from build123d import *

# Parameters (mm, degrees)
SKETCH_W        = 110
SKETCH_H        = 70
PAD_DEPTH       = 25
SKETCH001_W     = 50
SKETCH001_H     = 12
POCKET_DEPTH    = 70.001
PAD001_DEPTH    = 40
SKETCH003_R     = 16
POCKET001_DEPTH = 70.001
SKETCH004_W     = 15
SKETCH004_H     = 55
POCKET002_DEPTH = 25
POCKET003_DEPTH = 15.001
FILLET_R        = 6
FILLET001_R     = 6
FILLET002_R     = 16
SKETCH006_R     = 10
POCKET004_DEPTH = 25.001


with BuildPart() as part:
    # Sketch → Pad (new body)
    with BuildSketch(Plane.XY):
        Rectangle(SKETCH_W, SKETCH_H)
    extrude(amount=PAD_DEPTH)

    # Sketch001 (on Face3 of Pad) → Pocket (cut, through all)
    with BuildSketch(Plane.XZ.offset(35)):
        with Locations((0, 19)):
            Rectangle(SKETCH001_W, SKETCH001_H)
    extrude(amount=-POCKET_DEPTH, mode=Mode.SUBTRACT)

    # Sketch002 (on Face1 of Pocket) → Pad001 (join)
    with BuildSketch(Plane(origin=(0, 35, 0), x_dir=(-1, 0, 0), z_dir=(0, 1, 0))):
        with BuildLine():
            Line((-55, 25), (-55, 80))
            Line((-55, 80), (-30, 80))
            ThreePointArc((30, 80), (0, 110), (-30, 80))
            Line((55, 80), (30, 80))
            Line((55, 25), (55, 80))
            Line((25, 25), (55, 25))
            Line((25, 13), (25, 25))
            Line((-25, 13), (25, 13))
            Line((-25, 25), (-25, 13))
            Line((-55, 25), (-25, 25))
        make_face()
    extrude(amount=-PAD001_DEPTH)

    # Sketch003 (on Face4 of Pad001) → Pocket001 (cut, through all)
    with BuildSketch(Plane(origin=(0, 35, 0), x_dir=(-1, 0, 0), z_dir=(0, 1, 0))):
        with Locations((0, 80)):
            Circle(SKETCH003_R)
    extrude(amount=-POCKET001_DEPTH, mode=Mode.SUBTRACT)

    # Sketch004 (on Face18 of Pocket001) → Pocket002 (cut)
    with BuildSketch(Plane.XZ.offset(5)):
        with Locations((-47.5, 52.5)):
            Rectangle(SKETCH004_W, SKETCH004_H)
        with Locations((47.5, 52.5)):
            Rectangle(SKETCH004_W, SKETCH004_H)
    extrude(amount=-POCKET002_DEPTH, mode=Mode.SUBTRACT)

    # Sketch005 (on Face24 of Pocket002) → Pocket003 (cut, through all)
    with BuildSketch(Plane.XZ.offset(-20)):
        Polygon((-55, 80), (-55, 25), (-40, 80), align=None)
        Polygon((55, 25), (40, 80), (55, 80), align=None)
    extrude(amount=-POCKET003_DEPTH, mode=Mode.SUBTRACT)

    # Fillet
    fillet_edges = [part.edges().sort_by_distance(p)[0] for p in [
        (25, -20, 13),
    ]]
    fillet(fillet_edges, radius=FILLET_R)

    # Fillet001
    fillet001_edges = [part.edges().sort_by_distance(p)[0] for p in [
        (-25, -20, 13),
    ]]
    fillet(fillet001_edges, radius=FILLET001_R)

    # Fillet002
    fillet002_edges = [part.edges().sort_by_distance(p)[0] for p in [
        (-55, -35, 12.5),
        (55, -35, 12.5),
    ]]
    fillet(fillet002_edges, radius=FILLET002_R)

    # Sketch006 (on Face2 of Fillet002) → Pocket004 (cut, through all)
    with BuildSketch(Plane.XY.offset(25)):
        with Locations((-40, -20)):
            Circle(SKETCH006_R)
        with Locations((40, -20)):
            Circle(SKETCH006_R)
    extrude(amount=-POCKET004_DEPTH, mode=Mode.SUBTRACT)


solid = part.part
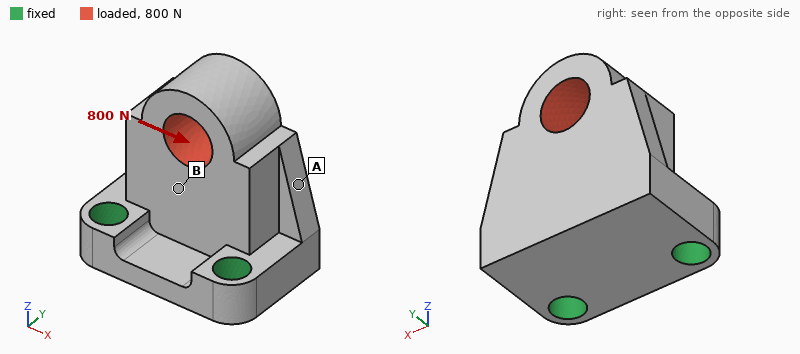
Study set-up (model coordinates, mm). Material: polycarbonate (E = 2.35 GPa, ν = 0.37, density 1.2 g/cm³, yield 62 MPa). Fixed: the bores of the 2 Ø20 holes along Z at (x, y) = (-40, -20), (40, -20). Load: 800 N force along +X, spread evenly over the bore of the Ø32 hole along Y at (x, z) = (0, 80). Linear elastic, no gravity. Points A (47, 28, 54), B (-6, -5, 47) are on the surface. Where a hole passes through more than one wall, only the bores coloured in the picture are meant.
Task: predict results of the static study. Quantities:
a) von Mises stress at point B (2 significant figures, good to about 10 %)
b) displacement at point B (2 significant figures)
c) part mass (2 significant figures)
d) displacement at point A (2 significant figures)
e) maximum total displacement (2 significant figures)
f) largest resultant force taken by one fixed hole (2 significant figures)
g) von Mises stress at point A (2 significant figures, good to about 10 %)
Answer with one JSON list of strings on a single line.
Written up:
["1.2 MPa", "0.051 mm", "440 g", "0.076 mm", "0.14 mm", "810 N", "0.61 MPa"]
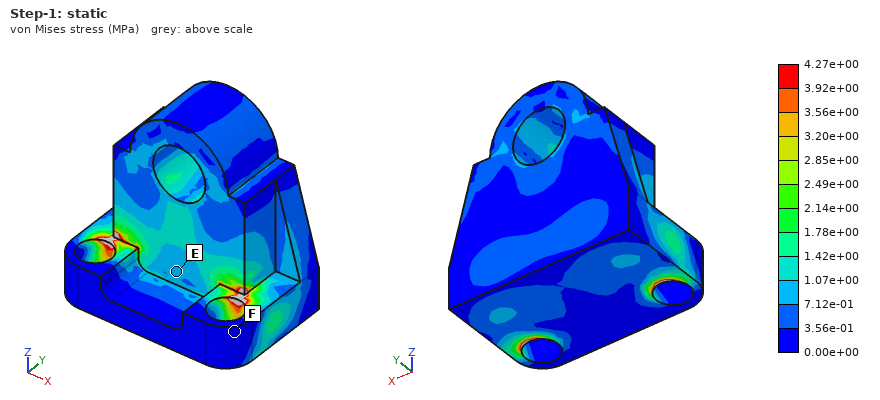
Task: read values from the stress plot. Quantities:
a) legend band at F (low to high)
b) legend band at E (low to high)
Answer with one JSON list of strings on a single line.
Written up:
["0.00e+00 to 3.56e-01 MPa", "7.12e-01 to 1.07e+00 MPa"]
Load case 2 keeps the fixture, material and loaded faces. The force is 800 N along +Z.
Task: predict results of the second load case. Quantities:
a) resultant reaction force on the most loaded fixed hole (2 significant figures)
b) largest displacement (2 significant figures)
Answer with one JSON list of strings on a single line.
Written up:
["400 N", "0.17 mm"]
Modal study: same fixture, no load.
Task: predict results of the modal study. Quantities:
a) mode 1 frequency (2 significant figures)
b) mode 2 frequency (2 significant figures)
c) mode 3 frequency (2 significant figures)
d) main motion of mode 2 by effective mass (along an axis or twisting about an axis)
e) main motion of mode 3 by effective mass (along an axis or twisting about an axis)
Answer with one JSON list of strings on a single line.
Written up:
["510 Hz", "1100 Hz", "1700 Hz", "along X", "along Z"]
